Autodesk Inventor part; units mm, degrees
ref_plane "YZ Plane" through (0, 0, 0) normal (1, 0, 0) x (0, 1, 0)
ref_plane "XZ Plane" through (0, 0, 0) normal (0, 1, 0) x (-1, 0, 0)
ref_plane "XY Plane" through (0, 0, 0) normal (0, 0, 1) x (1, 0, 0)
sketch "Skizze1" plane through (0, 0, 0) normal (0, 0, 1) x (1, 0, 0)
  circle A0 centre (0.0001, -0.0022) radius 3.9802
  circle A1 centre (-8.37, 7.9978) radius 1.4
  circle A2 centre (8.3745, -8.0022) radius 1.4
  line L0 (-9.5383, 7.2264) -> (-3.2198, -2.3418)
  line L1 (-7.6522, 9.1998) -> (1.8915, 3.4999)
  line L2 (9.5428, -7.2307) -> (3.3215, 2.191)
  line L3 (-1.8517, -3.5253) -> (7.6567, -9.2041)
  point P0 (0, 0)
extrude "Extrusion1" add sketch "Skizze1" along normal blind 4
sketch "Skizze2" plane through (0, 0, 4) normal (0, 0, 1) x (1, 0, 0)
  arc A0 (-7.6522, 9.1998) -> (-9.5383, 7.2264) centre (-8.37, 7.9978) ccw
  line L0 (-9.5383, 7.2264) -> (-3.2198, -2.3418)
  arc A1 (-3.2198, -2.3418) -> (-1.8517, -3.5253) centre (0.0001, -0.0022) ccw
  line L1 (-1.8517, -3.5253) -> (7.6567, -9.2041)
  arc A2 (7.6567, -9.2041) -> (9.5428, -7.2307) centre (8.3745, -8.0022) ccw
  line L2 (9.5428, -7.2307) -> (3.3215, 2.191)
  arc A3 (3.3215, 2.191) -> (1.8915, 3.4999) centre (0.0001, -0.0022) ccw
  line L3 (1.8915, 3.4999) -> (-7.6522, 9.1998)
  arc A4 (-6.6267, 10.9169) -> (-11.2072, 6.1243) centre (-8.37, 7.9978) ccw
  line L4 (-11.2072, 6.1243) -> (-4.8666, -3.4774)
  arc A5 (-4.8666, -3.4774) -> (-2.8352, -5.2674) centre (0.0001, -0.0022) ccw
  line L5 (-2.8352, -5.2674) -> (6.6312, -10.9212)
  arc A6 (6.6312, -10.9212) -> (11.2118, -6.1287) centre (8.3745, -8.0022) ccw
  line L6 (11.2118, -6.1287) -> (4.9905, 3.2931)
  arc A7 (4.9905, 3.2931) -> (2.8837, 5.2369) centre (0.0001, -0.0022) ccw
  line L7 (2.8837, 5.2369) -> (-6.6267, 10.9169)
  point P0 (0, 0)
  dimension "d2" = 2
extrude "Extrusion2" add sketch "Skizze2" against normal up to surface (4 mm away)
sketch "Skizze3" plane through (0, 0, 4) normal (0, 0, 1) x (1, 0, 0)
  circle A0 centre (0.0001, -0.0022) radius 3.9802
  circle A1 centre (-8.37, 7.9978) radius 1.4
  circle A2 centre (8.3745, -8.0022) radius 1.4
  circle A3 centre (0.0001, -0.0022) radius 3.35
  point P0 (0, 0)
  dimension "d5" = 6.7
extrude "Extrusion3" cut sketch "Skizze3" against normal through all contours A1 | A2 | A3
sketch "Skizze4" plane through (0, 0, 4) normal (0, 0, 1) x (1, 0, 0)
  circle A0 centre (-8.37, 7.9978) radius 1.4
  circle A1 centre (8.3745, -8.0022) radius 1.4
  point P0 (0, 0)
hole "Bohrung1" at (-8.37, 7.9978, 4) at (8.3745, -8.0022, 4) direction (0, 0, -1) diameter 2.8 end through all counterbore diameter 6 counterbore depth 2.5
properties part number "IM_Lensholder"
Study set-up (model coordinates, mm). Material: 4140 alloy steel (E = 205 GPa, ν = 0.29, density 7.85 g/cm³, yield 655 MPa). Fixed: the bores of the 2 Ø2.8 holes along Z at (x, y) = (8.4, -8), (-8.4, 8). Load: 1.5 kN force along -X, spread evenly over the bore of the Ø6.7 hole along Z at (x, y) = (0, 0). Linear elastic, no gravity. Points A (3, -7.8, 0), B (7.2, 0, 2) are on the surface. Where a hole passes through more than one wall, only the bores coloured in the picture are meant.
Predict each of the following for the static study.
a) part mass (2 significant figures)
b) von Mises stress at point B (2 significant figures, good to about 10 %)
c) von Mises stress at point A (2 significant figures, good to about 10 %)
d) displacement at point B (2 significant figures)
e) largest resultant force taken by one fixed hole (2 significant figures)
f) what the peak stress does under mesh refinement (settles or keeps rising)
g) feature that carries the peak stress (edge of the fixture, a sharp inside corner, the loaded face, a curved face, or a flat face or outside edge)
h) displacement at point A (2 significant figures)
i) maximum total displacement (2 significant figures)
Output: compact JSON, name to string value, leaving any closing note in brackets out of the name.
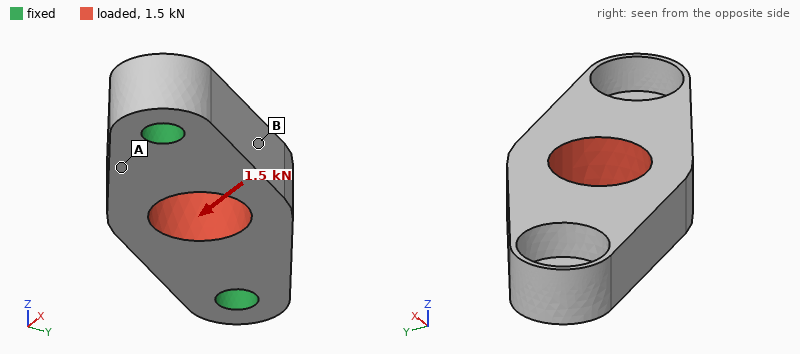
{"part mass": "5.8 g", "von Mises stress at point B": "31 MPa", "von Mises stress at point A": "73 MPa", "displacement at point B": "7.3 µm", "largest resultant force taken by one fixed hole": "750 N", "what the peak stress does under mesh refinement": "keeps rising", "feature that carries the peak stress": "edge of the fixture", "displacement at point A": "4.0 µm", "maximum total displacement": "10 µm"}
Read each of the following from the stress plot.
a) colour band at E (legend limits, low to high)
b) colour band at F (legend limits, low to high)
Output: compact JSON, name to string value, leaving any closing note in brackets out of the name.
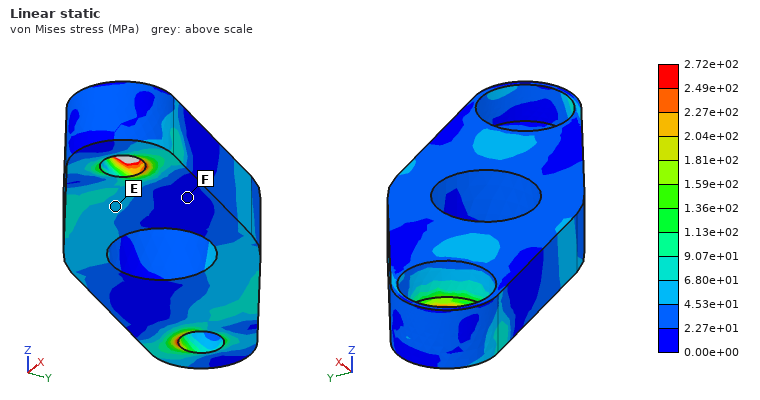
{"colour band at E": "4.53e+01 to 6.80e+01 MPa", "colour band at F": "0.00e+00 to 2.27e+01 MPa"}
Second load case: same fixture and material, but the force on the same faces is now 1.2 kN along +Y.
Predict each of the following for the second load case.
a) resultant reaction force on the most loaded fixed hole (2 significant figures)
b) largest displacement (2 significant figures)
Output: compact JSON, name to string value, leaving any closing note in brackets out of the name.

{"resultant reaction force on the most loaded fixed hole": "600 N", "largest displacement": "8.7 µm"}
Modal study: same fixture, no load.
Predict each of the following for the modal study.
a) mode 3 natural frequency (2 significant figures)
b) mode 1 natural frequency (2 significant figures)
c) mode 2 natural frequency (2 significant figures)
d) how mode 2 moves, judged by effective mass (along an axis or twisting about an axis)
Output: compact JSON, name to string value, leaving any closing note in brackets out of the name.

{"mode 3 natural frequency": "44 kHz", "mode 1 natural frequency": "21 kHz", "mode 2 natural frequency": "23 kHz", "how mode 2 moves, judged by effective mass": "along Z"}
